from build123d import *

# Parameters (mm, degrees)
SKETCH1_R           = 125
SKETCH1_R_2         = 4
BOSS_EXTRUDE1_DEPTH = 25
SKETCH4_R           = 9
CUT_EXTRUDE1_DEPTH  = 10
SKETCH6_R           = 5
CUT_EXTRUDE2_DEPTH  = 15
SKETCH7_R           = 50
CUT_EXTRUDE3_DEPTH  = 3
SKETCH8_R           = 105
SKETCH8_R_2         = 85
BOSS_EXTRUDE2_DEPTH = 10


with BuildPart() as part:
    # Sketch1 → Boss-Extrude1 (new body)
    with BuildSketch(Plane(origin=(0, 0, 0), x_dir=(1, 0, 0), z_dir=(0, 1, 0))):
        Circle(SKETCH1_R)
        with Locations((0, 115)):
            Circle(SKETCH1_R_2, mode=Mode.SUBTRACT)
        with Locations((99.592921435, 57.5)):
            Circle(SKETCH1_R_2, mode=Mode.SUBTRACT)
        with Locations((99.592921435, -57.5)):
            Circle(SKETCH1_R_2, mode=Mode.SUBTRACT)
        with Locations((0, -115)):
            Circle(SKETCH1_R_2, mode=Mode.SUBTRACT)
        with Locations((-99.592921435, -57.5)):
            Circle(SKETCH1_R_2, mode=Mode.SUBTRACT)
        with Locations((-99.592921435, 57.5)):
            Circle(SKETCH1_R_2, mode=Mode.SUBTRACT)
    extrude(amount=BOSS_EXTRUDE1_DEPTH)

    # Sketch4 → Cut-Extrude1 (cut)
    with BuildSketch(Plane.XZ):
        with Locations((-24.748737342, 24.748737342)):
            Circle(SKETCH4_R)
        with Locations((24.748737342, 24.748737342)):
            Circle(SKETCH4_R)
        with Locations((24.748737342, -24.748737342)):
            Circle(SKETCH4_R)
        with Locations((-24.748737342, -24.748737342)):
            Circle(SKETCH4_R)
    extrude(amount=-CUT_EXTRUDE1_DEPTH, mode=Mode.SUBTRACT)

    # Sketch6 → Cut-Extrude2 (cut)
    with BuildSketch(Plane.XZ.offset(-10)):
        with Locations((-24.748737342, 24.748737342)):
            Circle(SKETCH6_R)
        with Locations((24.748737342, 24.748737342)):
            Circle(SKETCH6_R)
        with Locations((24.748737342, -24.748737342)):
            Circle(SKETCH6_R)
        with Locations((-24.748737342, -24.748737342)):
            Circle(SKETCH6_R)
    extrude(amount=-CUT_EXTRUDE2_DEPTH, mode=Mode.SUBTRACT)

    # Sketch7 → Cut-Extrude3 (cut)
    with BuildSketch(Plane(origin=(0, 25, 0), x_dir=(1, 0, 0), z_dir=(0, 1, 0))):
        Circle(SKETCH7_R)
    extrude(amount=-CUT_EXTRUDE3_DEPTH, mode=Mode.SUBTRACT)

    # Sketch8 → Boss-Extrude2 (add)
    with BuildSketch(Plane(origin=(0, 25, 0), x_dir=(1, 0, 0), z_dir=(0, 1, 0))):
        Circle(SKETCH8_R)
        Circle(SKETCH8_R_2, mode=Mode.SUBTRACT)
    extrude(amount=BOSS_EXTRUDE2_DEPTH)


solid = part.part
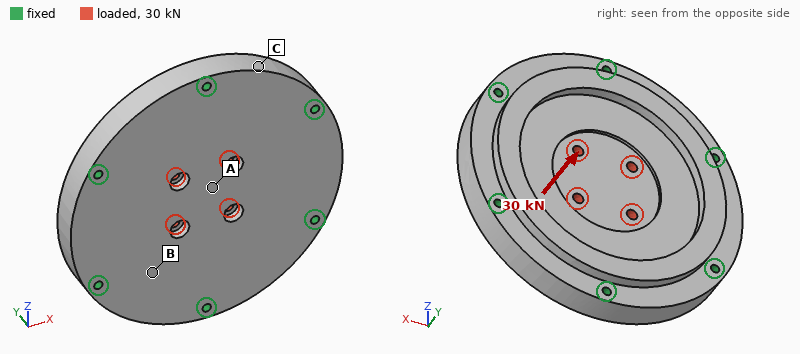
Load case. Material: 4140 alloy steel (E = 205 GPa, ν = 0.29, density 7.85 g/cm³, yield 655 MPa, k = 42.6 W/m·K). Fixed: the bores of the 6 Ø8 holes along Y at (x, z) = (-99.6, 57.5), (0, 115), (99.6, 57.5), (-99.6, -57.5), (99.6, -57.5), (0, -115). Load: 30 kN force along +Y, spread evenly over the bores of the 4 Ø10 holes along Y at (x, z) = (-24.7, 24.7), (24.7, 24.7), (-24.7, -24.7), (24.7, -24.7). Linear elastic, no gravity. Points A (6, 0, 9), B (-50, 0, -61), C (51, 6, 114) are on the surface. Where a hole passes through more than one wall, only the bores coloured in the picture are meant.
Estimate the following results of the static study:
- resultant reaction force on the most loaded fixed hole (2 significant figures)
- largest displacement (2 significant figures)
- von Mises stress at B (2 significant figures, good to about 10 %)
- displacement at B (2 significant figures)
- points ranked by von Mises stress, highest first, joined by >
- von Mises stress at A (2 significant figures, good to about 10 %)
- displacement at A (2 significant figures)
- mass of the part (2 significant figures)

5.0 kN
39 µm
16 MPa
13 µm
A > B > C
31 MPa
38 µm
10 kg
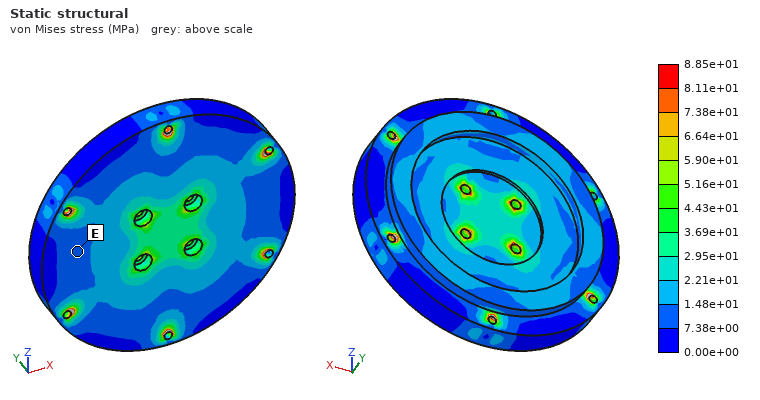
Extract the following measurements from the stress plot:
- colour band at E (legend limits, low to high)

7.38e+00 to 1.48e+01 MPa
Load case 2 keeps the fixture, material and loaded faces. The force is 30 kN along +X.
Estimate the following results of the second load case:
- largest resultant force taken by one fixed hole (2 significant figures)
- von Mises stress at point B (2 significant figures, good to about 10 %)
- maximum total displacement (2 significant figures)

6.3 kN
3.0 MPa
4.1 µm
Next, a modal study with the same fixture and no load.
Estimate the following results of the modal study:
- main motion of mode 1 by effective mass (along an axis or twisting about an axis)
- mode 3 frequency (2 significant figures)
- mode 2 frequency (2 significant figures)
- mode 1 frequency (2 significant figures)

along Y
5900 Hz
5900 Hz
3100 Hz
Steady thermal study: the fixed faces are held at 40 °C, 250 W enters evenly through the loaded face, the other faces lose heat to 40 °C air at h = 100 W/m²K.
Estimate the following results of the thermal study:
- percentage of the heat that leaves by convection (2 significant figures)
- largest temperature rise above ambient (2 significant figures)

61 %
56 K
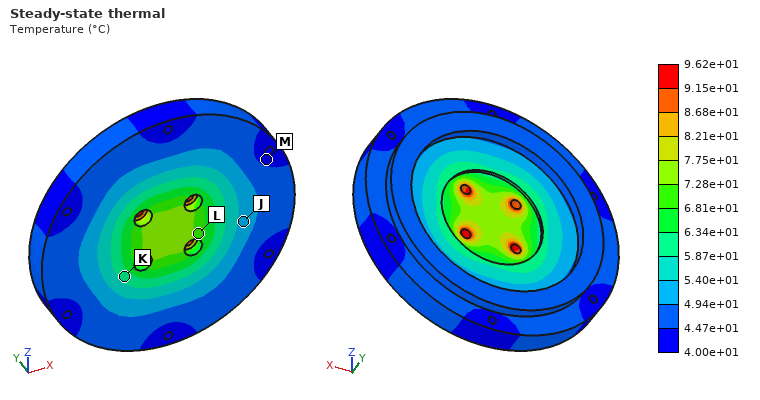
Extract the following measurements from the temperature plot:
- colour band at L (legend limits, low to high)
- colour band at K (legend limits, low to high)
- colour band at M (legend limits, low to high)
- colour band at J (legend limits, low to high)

6.81e+01 to 7.28e+01 °C
5.87e+01 to 6.34e+01 °C
4.00e+01 to 4.47e+01 °C
4.94e+01 to 5.40e+01 °C
